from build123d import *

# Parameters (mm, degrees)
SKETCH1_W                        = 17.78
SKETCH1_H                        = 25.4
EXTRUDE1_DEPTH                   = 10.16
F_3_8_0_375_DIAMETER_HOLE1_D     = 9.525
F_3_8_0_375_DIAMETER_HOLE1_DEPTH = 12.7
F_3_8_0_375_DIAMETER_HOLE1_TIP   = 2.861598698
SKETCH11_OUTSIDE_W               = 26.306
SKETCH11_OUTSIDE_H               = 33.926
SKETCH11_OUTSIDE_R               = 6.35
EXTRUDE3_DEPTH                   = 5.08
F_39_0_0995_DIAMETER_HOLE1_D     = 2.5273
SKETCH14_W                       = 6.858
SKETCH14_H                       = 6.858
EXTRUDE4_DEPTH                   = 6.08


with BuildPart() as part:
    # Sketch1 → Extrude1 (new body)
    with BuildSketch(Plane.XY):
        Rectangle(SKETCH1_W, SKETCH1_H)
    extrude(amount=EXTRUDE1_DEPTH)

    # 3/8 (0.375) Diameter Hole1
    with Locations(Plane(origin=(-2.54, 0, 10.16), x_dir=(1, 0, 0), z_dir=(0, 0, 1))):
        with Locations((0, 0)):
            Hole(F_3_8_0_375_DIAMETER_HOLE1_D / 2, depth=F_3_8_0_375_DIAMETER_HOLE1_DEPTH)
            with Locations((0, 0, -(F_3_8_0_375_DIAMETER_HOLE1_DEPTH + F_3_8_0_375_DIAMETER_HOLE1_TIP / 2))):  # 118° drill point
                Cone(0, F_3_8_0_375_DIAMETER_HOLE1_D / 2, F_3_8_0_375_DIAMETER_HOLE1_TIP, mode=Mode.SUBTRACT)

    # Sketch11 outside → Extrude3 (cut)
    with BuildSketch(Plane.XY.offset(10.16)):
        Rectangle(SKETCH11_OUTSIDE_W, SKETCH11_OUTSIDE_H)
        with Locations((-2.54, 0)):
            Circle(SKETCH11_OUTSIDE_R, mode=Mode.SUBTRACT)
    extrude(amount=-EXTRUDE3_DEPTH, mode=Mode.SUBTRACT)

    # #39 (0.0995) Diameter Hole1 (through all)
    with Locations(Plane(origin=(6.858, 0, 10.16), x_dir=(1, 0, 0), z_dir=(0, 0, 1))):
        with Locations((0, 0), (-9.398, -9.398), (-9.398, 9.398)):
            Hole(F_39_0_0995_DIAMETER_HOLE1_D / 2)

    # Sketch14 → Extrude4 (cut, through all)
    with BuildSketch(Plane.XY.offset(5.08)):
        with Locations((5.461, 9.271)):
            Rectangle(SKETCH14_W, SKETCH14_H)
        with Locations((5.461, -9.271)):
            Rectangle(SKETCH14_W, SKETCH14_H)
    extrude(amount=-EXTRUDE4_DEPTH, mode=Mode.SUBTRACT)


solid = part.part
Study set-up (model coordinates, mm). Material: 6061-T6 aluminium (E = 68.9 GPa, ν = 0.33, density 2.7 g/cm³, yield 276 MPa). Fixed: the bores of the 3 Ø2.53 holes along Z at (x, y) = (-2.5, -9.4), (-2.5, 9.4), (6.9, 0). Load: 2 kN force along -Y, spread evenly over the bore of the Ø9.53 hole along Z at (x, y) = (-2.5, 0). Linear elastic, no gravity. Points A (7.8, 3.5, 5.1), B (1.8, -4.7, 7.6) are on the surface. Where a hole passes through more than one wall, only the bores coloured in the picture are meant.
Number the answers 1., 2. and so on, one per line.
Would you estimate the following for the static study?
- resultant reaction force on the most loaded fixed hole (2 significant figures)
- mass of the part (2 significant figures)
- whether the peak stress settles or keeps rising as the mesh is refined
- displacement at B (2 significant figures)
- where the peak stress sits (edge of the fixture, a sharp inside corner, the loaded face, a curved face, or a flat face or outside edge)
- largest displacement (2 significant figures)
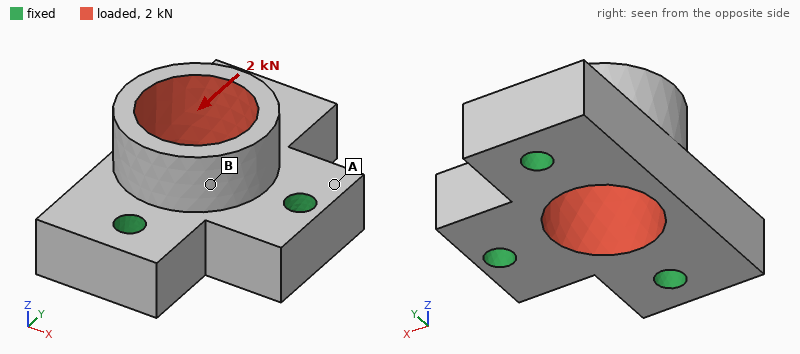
1. 880 N
2. 4.5 g
3. keeps rising
4. 5.5 µm
5. edge of the fixture
6. 9.3 µm
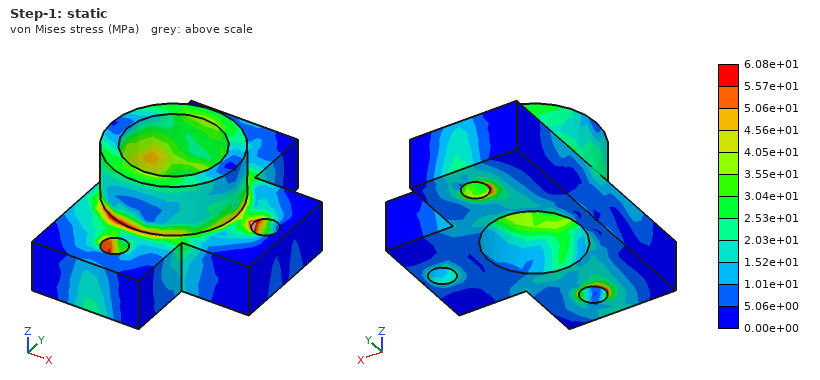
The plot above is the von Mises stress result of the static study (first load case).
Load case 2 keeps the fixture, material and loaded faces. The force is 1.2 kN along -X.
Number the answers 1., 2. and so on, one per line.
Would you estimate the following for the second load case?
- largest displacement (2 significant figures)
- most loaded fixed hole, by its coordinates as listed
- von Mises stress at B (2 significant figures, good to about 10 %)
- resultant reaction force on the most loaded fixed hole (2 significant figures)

1. 13 µm
2. (6.9, 0)
3. 17 MPa
4. 510 N
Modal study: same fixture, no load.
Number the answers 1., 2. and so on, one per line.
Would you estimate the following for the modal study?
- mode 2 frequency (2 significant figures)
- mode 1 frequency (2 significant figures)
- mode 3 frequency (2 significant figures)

1. 53 kHz
2. 40 kHz
3. 68 kHz
